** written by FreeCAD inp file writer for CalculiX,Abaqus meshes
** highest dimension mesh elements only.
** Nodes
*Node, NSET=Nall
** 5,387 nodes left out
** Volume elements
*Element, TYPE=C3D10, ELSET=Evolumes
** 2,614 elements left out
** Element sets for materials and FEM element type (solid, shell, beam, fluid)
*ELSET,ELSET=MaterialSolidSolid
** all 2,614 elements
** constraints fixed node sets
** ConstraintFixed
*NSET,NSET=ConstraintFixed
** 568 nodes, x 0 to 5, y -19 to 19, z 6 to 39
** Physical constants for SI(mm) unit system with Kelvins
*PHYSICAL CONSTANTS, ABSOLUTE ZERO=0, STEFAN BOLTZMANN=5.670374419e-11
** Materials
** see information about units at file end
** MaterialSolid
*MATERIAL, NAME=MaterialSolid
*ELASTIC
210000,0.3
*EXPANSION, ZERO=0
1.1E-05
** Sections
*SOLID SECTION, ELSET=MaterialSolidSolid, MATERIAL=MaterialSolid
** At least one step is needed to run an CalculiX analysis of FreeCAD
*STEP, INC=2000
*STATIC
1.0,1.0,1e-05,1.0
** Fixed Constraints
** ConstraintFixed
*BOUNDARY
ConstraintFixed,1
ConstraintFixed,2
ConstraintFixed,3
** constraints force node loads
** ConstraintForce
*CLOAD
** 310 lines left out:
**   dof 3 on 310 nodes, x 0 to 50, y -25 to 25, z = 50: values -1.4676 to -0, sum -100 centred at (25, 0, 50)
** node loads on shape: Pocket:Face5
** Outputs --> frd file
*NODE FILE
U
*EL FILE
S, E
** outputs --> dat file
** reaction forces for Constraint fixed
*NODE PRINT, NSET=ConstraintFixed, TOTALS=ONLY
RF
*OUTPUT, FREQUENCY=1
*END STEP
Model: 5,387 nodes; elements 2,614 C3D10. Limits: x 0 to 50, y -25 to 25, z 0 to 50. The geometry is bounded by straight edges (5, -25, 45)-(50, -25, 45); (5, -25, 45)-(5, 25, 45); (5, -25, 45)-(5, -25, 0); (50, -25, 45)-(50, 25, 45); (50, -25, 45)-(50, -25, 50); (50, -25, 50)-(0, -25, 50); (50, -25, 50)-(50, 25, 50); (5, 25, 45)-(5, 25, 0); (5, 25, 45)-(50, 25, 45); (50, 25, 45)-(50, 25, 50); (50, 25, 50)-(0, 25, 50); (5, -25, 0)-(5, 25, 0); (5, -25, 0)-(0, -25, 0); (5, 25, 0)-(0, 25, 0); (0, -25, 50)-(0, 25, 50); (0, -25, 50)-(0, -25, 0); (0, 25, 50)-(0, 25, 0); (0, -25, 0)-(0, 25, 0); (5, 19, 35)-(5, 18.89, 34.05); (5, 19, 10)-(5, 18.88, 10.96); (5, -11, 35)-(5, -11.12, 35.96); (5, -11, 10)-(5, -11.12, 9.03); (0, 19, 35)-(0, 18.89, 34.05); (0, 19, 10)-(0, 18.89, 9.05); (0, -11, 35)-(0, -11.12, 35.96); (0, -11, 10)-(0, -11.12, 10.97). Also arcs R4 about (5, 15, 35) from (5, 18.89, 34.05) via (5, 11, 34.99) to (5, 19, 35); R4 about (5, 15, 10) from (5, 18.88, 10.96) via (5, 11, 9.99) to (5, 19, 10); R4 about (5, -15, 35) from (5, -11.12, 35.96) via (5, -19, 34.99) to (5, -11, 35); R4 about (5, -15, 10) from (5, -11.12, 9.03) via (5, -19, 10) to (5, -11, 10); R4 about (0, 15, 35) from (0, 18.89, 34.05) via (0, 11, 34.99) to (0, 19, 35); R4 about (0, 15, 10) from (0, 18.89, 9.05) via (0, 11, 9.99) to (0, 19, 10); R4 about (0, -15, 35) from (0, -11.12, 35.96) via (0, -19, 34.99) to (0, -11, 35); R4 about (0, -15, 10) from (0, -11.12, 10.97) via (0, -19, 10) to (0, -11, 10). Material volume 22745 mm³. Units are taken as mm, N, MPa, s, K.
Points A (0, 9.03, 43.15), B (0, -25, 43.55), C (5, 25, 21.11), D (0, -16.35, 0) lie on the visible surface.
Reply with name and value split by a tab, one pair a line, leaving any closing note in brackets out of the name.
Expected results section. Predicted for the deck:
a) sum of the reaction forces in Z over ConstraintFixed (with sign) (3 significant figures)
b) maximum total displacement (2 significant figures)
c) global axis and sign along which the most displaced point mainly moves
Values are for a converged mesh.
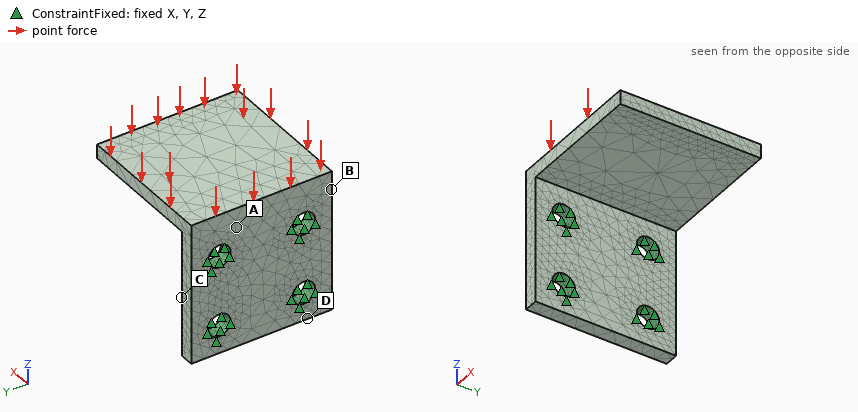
sum of the reaction forces in Z over ConstraintFixed (with sign)	100 N
maximum total displacement	0.019 mm
global axis and sign along which the most displaced point mainly moves	-Z
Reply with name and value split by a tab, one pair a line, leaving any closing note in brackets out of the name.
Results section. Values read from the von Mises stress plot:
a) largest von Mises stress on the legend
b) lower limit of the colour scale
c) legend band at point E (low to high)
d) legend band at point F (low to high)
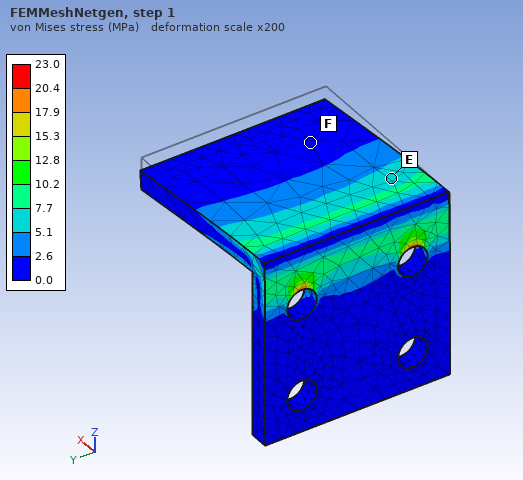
largest von Mises stress on the legend	23.0 MPa
lower limit of the colour scale	0.0 MPa
legend band at point E	5.1 to 7.7 MPa
legend band at point F	0.0 to 2.6 MPa
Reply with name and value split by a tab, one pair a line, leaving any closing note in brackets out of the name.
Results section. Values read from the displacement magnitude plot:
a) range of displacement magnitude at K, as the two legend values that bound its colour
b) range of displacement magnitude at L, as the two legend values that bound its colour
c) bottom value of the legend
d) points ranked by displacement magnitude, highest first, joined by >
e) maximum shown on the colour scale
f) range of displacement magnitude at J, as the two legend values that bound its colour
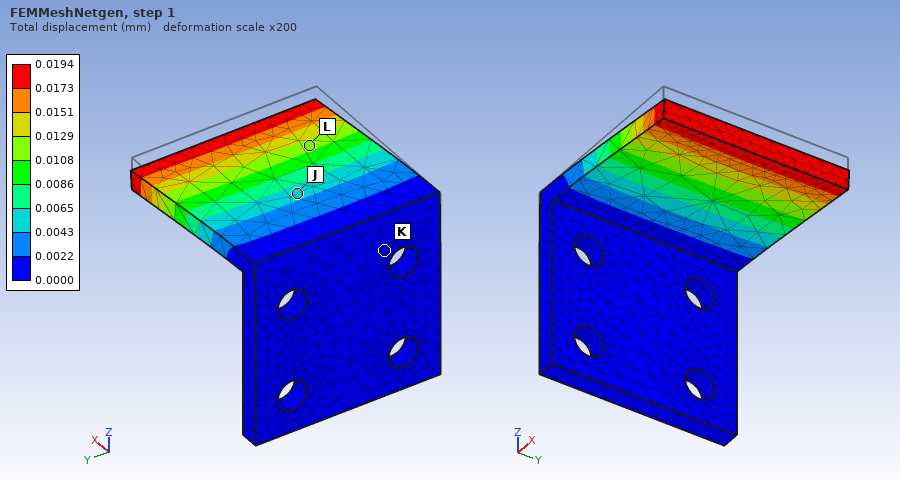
range of displacement magnitude at K, as the two legend values that bound its colour	0.0000 to 0.0022 mm
range of displacement magnitude at L, as the two legend values that bound its colour	0.0108 to 0.0129 mm
bottom value of the legend	0.0000 mm
points ranked by displacement magnitude, highest first, joined by >	L > J > K
maximum shown on the colour scale	0.0194 mm
range of displacement magnitude at J, as the two legend values that bound its colour	0.0043 to 0.0065 mm
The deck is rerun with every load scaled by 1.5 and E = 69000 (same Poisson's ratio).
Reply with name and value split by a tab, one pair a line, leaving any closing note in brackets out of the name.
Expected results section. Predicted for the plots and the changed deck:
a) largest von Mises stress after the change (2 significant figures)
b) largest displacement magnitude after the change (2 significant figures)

largest von Mises stress after the change	34 MPa
largest displacement magnitude after the change	0.089 mm
